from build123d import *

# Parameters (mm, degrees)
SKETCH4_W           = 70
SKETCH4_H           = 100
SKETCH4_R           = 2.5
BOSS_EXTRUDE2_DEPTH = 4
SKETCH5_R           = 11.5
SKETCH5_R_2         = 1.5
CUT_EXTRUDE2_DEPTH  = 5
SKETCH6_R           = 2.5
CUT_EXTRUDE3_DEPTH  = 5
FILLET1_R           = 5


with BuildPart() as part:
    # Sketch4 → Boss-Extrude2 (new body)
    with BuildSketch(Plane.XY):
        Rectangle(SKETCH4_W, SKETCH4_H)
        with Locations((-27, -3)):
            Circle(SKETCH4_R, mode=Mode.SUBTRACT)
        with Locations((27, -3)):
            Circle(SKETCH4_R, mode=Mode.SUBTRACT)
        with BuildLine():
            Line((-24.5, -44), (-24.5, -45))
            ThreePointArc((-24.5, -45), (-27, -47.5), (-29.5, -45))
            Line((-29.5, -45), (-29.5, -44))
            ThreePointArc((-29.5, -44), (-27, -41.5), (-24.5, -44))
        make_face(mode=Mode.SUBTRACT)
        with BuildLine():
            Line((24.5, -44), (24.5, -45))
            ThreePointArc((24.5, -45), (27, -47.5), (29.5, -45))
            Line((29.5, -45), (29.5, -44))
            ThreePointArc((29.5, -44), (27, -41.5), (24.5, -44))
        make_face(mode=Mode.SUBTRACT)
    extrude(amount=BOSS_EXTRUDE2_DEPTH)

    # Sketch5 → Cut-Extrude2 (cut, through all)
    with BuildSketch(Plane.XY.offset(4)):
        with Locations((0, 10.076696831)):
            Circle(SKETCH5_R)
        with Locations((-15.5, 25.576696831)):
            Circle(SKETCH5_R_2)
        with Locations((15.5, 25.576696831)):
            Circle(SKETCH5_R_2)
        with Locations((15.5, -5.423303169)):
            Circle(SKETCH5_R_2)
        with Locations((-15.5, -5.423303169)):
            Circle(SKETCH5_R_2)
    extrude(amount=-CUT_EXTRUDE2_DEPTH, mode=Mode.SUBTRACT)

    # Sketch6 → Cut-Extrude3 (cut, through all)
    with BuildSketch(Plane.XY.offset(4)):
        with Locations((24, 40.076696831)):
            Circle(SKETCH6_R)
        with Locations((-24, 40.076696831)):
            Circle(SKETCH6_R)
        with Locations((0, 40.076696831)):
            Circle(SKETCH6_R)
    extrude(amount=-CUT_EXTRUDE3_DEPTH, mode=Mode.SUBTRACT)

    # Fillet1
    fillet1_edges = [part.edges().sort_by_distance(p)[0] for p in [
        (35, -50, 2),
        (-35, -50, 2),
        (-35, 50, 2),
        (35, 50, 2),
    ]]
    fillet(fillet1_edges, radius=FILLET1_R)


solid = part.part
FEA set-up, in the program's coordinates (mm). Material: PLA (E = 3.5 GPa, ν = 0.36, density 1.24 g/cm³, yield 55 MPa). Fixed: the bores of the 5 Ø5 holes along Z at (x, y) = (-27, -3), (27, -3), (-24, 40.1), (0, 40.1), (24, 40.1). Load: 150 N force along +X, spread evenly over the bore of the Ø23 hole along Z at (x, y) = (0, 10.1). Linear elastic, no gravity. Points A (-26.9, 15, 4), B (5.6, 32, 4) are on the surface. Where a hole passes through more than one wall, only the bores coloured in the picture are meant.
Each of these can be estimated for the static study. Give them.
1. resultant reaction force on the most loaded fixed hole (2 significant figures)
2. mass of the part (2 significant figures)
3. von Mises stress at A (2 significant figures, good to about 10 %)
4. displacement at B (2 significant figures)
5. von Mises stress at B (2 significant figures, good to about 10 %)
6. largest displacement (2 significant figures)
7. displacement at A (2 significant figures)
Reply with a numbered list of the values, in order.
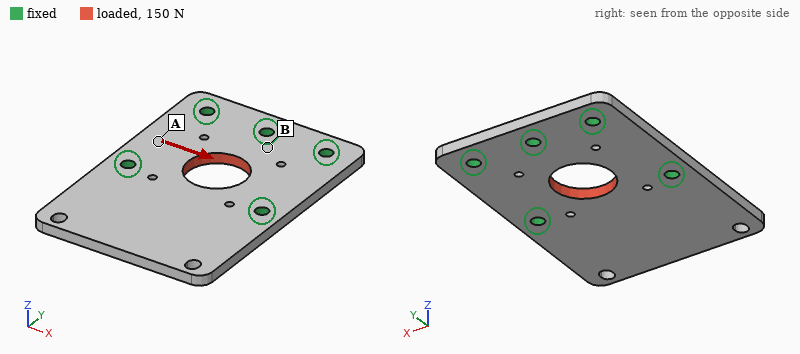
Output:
1. 47 N
2. 32 g
3. 0.15 MPa
4. 1.6 µm
5. 0.40 MPa
6. 5.0 µm
7. 3.6 µm
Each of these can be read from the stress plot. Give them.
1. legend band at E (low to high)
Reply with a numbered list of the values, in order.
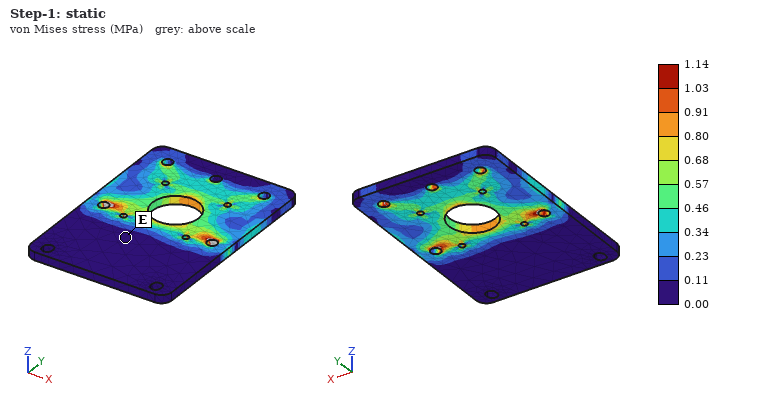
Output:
1. 0.00 to 0.11 MPa
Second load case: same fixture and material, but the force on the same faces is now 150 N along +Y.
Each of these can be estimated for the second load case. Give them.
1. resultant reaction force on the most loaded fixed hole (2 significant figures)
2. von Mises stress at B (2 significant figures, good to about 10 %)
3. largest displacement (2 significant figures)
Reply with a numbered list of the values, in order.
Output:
1. 38 N
2. 0.41 MPa
3. 5.7 µm
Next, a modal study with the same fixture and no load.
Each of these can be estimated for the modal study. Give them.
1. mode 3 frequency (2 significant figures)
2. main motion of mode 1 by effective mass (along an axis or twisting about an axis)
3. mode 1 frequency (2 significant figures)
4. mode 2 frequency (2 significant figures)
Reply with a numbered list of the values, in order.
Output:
1. 2000 Hz
2. along Z
3. 450 Hz
4. 960 Hz
